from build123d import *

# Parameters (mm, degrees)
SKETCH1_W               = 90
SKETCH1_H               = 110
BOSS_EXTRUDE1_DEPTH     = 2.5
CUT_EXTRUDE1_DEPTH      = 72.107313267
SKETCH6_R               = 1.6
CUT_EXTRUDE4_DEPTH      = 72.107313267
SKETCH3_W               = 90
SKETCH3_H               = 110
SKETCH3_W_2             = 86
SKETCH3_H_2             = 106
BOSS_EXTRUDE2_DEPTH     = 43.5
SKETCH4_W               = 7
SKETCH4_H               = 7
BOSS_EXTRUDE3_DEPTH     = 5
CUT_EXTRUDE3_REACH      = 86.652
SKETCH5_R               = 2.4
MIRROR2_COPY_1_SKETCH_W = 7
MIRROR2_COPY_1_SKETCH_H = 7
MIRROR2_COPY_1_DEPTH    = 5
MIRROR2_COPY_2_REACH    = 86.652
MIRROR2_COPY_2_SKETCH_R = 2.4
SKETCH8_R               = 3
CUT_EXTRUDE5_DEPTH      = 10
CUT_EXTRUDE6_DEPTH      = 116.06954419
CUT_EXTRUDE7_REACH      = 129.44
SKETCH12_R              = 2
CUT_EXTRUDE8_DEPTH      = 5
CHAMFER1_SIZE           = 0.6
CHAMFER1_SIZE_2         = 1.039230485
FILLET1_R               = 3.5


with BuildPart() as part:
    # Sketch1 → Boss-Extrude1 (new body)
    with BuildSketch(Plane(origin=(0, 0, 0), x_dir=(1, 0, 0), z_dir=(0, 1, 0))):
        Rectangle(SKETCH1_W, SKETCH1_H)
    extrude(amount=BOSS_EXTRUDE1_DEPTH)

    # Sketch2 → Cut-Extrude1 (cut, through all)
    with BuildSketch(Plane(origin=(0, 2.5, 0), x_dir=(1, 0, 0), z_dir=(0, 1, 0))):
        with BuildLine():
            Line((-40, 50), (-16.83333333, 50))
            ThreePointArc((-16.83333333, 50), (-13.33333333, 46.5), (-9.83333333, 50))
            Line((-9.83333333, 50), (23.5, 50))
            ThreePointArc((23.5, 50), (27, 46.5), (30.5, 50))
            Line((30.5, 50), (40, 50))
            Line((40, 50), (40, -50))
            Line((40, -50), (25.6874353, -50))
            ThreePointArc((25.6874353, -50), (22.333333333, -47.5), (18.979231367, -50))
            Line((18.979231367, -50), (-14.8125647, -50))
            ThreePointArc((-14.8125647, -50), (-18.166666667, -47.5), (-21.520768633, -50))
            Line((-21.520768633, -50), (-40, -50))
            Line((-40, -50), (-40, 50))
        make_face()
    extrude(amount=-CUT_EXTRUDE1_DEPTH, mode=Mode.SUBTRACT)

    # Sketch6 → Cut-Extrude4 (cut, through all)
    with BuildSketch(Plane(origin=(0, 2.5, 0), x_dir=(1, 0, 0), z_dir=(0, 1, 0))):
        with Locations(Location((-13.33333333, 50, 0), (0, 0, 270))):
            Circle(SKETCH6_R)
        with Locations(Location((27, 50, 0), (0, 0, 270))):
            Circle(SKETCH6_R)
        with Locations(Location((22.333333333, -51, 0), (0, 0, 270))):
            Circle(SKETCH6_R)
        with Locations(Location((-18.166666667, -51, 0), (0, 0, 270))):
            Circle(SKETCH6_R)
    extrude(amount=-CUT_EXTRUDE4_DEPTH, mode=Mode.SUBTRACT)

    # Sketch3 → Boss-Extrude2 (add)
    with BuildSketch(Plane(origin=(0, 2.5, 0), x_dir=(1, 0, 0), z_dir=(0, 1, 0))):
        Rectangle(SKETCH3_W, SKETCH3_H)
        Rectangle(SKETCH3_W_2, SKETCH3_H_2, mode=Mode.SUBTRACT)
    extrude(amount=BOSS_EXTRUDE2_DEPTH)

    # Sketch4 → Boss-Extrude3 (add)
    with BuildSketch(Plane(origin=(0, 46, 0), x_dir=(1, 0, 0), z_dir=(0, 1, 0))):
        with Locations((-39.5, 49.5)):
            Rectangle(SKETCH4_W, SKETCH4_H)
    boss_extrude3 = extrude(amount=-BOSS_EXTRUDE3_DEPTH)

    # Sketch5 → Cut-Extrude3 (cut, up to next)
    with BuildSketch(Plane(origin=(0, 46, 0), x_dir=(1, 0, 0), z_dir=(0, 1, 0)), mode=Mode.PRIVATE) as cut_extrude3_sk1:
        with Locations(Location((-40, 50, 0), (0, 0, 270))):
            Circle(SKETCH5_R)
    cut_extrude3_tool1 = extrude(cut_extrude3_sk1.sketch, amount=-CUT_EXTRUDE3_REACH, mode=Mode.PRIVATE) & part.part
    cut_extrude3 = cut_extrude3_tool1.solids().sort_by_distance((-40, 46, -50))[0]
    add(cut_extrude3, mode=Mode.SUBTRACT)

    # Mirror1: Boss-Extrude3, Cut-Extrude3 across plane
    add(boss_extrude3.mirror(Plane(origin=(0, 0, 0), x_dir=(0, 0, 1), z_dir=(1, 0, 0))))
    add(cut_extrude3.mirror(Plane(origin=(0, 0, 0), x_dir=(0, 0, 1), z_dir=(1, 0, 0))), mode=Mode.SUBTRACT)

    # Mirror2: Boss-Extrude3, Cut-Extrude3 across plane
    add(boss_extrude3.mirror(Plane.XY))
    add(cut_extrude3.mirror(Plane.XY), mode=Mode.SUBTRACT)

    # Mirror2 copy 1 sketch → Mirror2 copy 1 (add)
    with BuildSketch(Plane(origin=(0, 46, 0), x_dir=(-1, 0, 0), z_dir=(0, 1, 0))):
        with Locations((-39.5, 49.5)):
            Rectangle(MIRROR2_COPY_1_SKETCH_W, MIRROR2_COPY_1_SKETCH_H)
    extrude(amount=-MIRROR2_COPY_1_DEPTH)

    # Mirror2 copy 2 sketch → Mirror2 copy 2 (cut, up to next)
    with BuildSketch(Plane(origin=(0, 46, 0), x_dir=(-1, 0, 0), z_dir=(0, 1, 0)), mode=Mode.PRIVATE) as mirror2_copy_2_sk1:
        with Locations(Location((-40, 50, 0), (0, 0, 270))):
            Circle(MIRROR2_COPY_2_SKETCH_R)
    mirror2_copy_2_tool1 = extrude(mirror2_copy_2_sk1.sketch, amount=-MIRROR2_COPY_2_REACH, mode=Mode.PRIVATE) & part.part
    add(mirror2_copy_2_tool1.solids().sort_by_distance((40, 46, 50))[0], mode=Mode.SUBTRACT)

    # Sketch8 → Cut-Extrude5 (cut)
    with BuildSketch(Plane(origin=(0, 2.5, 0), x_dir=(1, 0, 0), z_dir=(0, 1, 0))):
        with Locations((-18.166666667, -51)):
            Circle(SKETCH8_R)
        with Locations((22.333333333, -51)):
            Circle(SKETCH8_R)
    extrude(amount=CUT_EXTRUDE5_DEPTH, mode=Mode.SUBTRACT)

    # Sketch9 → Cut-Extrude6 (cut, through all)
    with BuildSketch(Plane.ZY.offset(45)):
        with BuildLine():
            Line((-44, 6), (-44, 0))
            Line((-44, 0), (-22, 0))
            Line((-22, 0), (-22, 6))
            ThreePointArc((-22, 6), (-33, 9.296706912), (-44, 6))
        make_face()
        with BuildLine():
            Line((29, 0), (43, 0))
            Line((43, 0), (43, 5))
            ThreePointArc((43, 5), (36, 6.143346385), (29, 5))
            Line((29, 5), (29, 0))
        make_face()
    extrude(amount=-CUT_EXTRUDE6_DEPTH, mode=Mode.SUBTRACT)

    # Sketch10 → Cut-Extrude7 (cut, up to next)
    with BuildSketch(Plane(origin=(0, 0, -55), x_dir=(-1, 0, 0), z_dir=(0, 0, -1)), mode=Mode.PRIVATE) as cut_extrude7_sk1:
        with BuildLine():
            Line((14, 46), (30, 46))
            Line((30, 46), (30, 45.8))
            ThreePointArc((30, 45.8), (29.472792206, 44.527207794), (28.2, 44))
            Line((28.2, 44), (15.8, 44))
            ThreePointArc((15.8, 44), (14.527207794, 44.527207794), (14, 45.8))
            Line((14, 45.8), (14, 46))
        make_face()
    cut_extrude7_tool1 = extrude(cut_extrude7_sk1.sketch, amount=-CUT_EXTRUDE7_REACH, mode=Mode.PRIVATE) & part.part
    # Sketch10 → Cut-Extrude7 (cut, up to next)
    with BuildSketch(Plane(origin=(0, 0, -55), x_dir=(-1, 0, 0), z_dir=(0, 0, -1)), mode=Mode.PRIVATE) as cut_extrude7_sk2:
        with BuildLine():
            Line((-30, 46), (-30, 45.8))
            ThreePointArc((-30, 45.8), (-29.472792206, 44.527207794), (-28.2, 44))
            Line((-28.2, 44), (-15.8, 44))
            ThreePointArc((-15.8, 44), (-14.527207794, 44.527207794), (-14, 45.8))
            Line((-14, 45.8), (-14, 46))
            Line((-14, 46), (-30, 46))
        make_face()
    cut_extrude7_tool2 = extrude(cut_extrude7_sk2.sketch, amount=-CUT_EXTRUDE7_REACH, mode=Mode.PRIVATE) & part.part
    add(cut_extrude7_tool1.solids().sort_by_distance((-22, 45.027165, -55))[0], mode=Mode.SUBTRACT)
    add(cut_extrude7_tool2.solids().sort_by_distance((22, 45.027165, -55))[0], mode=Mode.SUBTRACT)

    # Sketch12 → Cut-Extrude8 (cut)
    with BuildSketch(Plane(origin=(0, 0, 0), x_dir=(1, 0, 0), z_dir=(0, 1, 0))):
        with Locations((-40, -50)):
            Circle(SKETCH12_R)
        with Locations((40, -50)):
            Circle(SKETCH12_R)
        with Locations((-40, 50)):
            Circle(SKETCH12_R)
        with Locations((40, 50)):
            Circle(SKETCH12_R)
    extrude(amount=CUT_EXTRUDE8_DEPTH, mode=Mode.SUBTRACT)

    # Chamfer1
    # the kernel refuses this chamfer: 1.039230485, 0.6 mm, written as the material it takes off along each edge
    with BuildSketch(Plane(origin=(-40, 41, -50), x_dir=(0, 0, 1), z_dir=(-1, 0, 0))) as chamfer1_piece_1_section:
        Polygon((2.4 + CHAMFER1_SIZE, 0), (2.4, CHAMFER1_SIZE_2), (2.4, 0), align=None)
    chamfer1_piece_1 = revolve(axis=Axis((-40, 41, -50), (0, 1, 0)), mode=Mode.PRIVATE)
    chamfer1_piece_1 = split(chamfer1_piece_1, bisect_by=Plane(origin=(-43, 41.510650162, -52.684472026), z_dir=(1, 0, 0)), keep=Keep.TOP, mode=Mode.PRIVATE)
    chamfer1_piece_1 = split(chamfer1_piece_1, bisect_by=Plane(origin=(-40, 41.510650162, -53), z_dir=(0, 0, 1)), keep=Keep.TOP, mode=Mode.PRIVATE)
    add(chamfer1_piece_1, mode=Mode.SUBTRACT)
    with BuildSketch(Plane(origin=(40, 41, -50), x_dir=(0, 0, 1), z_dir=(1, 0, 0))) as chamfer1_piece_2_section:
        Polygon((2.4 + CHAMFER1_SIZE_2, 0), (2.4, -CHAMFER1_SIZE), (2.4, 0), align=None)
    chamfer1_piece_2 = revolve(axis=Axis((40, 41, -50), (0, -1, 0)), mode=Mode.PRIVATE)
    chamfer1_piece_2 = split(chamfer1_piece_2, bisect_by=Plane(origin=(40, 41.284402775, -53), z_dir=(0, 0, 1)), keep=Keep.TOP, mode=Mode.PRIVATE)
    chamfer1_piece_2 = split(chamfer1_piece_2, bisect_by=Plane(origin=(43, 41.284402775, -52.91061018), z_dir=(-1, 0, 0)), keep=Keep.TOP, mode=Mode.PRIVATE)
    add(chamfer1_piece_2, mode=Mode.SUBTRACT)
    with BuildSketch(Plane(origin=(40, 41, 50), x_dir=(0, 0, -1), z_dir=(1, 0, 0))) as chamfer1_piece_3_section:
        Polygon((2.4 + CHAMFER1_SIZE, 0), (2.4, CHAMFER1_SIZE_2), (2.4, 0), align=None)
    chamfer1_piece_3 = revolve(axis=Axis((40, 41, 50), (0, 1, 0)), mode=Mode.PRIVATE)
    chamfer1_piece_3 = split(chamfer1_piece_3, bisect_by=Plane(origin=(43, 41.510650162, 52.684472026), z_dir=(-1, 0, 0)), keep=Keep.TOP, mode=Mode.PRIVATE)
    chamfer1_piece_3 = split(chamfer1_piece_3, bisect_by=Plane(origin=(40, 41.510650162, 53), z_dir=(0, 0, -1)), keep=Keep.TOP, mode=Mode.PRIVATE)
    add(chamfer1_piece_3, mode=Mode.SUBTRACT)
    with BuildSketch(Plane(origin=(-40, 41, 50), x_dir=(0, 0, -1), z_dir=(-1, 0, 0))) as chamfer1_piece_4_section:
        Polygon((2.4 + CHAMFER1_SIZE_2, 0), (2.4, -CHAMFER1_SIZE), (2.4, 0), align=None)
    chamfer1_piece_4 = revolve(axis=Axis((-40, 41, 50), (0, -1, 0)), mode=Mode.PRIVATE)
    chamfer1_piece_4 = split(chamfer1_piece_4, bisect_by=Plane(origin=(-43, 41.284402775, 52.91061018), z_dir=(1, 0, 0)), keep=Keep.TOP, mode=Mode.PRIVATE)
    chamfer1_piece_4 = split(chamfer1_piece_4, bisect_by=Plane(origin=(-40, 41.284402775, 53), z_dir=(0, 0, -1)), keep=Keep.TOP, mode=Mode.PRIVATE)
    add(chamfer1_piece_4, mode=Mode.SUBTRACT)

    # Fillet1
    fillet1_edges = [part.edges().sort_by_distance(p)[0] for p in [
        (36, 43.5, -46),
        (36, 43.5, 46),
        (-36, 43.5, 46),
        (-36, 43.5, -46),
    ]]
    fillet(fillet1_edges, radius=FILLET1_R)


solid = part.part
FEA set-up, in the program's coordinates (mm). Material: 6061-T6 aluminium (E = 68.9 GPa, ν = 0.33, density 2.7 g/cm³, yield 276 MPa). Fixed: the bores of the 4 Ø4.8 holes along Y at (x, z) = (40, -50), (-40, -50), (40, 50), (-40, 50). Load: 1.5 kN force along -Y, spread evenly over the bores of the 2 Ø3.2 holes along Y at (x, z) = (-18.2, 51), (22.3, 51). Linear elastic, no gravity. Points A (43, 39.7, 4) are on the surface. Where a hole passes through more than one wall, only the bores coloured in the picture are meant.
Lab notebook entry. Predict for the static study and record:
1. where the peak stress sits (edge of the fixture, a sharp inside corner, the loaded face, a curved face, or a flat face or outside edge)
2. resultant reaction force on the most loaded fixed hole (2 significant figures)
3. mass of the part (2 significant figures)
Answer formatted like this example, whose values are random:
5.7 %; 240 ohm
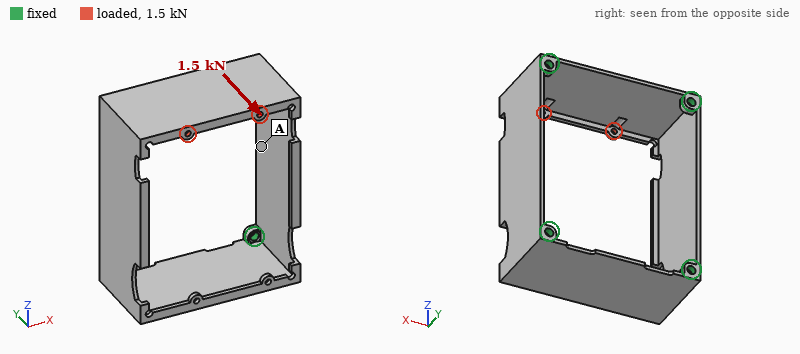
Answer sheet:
the loaded face; 850 N; 100 g
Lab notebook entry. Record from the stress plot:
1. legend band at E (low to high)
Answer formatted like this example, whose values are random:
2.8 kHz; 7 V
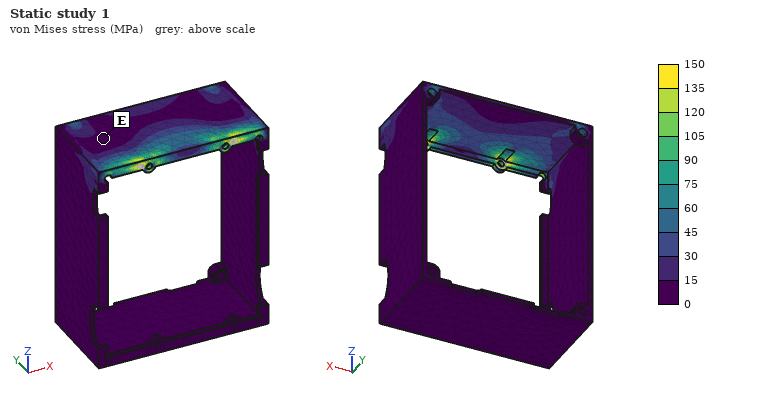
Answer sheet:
0 to 15 MPa
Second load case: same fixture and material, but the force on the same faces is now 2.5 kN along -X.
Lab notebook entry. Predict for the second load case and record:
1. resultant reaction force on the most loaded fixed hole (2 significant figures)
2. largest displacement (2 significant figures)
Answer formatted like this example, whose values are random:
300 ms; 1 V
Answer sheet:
1.8 kN; 77 µm
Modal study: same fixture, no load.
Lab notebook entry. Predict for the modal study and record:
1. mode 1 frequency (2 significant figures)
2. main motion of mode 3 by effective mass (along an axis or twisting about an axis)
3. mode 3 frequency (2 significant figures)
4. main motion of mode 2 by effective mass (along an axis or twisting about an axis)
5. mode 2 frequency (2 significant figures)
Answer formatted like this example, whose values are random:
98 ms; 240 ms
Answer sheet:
860 Hz; along Z; 1400 Hz; along X; 930 Hz
